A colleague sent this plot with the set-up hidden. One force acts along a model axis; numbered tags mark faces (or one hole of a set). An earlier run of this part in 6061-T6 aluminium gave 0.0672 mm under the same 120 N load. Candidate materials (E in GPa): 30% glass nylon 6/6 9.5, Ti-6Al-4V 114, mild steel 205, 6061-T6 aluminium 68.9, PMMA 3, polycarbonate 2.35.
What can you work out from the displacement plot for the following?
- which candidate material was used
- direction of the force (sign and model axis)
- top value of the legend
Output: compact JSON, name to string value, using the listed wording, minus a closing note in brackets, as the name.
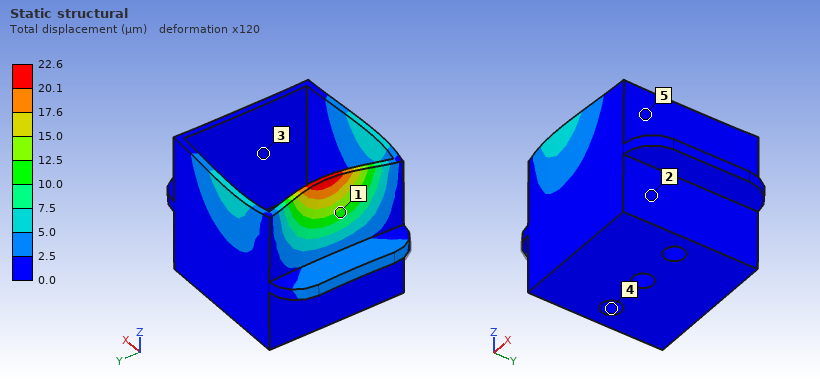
{"which candidate material was used": "mild steel", "direction of the force": "+X", "top value of the legend": "22.6 µm"}
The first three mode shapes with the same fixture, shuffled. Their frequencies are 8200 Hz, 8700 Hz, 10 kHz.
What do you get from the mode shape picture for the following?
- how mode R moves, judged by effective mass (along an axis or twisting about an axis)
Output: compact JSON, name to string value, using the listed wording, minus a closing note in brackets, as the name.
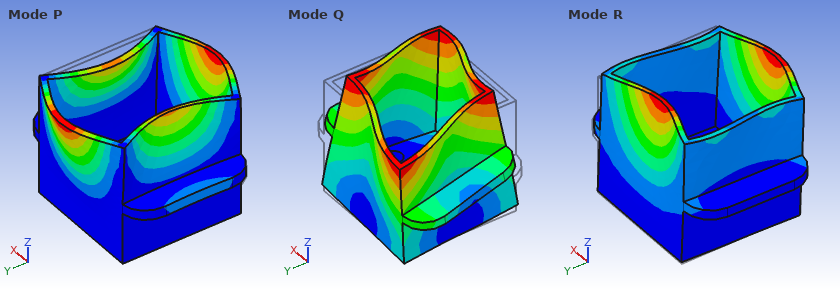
{"how mode R moves, judged by effective mass": "along Y"}
